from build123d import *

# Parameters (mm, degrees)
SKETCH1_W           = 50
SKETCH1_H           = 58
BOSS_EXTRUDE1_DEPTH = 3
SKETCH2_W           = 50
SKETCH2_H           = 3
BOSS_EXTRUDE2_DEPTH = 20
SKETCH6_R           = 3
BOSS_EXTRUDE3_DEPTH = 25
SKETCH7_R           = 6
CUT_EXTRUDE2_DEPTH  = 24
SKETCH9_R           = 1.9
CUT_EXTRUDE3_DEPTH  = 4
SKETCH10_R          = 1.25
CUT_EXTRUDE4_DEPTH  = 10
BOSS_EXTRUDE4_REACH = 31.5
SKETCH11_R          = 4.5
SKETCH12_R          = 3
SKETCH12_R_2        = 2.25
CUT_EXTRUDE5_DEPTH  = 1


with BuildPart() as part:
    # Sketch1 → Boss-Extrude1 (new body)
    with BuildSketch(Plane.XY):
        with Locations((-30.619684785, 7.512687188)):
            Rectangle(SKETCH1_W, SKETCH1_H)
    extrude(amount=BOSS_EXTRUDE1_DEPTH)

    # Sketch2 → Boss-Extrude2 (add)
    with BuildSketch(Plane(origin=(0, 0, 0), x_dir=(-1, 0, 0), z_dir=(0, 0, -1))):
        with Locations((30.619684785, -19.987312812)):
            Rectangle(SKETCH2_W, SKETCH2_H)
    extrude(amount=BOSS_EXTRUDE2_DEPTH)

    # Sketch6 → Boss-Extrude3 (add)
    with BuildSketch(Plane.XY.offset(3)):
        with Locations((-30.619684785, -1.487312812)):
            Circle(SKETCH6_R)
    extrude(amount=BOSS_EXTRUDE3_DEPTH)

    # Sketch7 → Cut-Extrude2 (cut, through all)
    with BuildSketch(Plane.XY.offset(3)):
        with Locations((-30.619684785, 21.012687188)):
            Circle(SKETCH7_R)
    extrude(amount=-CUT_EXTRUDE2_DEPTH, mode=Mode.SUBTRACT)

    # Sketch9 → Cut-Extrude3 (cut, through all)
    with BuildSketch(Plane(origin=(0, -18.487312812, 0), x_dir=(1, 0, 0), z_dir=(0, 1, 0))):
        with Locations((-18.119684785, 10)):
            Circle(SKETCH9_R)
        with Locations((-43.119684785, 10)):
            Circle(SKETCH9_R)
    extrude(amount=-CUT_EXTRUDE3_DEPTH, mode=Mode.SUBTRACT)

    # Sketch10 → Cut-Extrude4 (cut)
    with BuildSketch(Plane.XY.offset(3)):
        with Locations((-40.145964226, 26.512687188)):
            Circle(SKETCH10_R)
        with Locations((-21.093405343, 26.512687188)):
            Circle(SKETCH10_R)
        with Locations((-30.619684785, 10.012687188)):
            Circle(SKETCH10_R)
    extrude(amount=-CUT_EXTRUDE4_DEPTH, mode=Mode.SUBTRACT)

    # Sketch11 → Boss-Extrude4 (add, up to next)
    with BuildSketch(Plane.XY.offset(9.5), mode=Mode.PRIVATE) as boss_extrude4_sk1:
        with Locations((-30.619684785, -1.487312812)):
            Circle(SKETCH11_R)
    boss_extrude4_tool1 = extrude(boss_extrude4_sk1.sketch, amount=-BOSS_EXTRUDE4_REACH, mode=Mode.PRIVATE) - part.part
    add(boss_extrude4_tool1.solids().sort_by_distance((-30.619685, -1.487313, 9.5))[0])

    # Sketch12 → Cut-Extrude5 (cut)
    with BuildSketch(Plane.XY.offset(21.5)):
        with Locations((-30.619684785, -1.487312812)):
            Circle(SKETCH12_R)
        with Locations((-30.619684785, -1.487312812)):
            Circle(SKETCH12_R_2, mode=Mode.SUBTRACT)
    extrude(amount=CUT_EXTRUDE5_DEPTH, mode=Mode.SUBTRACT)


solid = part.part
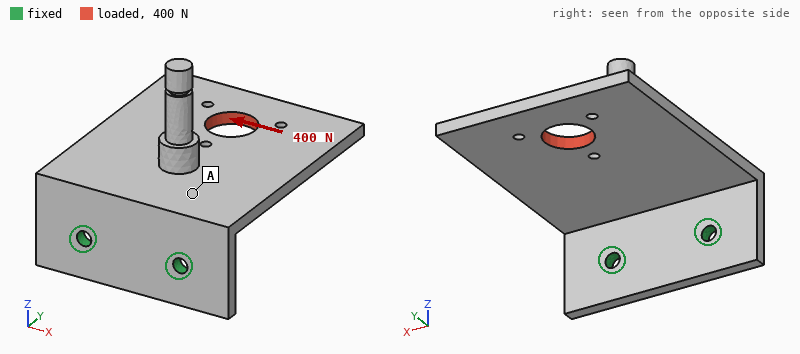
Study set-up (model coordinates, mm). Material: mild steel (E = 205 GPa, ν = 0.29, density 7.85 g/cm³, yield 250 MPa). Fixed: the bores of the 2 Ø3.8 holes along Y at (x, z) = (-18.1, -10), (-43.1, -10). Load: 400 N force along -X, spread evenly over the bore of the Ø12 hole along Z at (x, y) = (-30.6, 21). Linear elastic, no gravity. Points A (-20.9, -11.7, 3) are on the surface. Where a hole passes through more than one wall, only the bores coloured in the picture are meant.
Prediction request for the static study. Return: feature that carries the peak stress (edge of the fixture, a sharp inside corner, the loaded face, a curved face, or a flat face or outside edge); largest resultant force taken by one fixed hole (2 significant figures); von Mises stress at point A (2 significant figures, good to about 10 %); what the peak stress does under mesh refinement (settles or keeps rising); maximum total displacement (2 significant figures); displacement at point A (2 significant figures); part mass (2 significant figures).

edge of the fixture
610 N
18 MPa
keeps rising
87 µm
17 µm
96 g
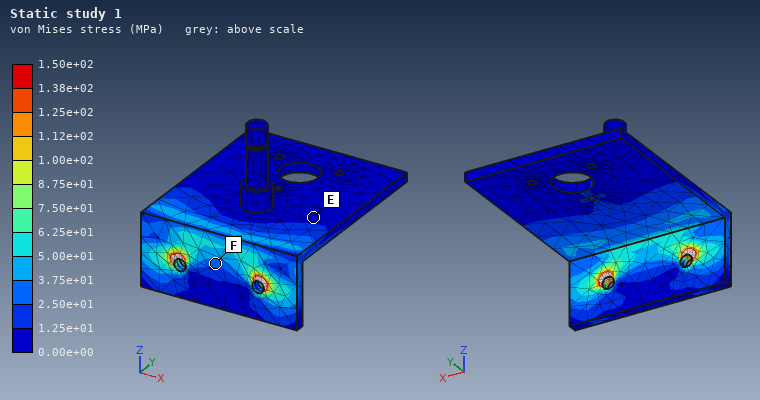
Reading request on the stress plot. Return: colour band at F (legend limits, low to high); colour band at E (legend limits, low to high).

2.50e+01 to 3.75e+01 MPa
0.00e+00 to 1.25e+01 MPa
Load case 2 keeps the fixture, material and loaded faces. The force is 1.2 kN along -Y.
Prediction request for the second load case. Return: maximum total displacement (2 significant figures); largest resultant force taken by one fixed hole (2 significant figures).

0.21 mm
600 N
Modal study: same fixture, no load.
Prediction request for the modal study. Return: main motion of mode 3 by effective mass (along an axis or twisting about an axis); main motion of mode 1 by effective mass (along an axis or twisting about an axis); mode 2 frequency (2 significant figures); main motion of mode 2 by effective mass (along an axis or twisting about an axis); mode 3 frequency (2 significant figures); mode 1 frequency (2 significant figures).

along X
along Z
1700 Hz
along X
2300 Hz
600 Hz
